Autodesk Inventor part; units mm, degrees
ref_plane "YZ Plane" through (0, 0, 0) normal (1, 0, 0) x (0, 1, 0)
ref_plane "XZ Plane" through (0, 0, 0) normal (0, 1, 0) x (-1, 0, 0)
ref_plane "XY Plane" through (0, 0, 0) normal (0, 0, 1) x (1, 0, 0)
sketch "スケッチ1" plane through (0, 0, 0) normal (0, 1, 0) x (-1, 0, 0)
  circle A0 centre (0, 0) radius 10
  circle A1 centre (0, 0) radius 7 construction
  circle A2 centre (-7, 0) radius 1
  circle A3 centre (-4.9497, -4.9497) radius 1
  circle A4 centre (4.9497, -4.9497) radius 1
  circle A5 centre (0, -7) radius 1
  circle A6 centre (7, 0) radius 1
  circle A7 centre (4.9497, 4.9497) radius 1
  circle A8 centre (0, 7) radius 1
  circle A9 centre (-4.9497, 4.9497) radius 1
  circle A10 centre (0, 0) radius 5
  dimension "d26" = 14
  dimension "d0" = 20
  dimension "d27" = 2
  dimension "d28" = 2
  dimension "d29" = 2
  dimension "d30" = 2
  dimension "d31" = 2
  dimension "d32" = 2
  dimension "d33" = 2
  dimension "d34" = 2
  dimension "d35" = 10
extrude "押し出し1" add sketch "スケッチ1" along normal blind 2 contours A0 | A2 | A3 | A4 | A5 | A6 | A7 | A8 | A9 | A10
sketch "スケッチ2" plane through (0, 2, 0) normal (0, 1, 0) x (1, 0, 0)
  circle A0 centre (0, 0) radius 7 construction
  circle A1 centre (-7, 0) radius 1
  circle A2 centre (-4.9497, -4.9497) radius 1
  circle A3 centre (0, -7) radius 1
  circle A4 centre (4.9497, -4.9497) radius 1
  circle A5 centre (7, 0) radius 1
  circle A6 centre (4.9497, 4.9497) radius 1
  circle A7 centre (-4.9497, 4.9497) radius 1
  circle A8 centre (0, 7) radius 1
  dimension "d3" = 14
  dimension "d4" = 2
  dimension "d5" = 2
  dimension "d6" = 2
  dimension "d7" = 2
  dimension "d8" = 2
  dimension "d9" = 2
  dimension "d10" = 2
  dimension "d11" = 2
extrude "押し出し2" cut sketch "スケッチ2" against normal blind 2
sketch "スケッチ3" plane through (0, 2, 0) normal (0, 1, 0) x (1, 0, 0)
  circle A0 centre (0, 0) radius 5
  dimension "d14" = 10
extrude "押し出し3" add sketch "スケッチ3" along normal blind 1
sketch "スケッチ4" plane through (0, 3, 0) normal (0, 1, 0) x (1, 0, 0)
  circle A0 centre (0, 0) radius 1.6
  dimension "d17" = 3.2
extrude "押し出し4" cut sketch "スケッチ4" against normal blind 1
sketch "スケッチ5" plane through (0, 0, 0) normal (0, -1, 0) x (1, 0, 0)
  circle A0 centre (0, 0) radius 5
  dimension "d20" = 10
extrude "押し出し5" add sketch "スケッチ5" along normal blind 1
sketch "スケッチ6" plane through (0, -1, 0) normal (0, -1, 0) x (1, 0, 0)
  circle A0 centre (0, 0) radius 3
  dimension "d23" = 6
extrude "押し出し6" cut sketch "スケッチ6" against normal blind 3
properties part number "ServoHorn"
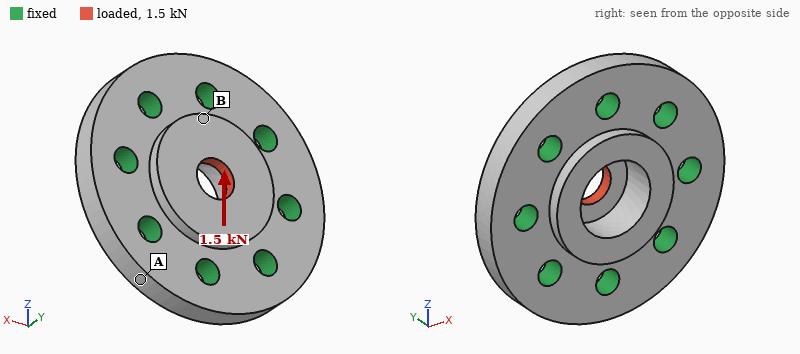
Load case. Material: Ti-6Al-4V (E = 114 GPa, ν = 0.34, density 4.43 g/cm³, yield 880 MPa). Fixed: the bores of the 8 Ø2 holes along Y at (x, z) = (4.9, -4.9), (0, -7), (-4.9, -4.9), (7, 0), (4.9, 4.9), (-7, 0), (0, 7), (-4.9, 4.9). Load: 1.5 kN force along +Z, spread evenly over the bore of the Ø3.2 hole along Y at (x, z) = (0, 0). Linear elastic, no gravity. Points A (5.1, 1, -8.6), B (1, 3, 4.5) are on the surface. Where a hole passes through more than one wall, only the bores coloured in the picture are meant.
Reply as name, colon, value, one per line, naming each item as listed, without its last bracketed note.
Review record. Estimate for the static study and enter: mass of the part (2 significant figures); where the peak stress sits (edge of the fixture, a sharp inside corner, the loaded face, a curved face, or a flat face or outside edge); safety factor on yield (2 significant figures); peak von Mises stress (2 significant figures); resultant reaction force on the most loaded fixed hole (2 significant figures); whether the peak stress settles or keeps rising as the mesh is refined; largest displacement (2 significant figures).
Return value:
mass of the part: 2.8 g
where the peak stress sits: the loaded face
safety factor on yield: 3.2
peak von Mises stress: 280 MPa
resultant reaction force on the most loaded fixed hole: 330 N
whether the peak stress settles or keeps rising as the mesh is refined: settles
largest displacement: 6.0 µm
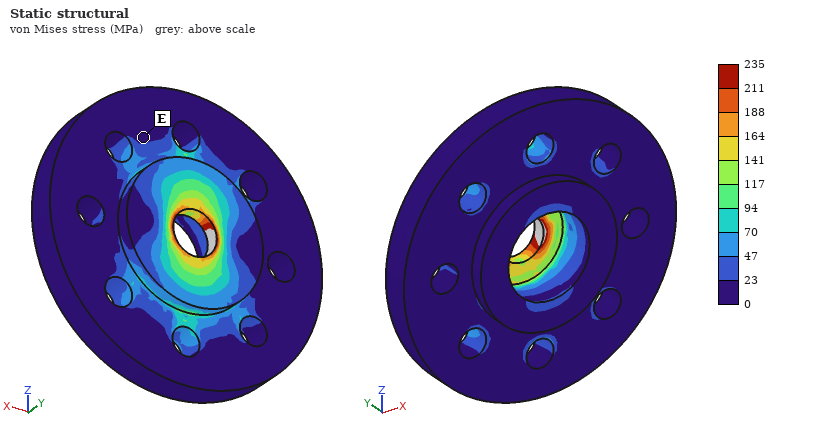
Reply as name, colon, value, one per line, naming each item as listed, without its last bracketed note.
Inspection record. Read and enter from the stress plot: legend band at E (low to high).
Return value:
legend band at E: 0 to 23 MPa
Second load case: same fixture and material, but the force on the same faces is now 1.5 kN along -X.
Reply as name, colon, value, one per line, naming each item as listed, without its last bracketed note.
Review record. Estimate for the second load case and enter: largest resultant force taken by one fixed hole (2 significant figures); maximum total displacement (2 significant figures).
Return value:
largest resultant force taken by one fixed hole: 330 N
maximum total displacement: 6.0 µm
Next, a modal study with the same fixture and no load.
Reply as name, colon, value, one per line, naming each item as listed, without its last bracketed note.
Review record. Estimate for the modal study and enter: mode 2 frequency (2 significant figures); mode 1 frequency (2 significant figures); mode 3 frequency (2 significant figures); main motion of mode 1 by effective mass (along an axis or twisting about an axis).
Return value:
mode 2 frequency: 150 kHz
mode 1 frequency: 120 kHz
mode 3 frequency: 150 kHz
main motion of mode 1 by effective mass: along Y
